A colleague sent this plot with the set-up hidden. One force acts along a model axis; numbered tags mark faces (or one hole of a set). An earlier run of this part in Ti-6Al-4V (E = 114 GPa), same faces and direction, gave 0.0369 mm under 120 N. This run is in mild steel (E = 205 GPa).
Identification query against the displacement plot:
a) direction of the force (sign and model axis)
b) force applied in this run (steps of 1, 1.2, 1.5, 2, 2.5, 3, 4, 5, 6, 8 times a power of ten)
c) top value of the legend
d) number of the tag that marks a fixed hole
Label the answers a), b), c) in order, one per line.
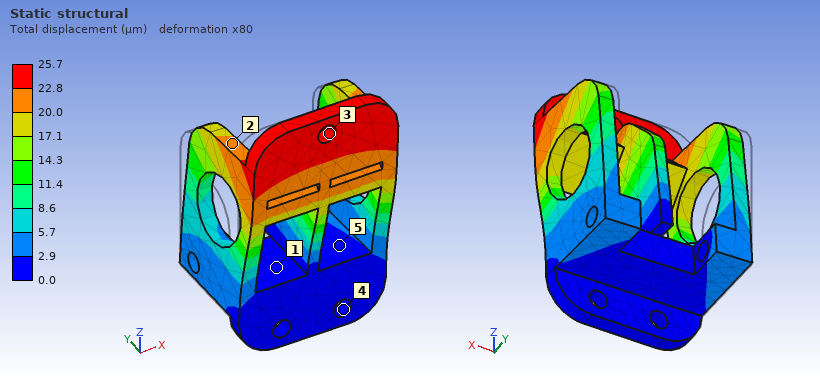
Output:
a) +X
b) 150 N
c) 25.7 µm
d) 4
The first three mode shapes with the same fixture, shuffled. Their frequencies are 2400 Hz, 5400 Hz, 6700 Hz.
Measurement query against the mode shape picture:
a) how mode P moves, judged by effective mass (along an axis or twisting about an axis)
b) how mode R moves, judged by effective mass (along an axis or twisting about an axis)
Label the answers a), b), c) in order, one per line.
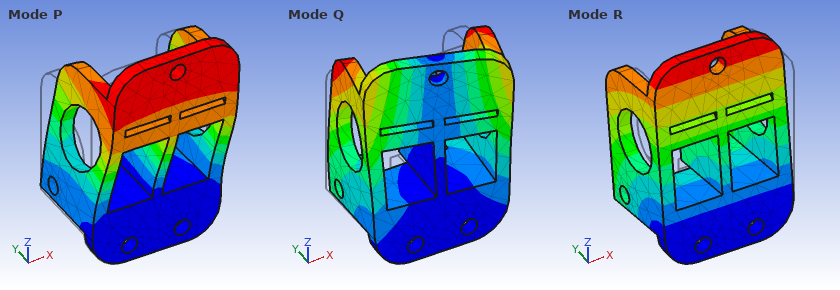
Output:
a) along X
b) along Y
